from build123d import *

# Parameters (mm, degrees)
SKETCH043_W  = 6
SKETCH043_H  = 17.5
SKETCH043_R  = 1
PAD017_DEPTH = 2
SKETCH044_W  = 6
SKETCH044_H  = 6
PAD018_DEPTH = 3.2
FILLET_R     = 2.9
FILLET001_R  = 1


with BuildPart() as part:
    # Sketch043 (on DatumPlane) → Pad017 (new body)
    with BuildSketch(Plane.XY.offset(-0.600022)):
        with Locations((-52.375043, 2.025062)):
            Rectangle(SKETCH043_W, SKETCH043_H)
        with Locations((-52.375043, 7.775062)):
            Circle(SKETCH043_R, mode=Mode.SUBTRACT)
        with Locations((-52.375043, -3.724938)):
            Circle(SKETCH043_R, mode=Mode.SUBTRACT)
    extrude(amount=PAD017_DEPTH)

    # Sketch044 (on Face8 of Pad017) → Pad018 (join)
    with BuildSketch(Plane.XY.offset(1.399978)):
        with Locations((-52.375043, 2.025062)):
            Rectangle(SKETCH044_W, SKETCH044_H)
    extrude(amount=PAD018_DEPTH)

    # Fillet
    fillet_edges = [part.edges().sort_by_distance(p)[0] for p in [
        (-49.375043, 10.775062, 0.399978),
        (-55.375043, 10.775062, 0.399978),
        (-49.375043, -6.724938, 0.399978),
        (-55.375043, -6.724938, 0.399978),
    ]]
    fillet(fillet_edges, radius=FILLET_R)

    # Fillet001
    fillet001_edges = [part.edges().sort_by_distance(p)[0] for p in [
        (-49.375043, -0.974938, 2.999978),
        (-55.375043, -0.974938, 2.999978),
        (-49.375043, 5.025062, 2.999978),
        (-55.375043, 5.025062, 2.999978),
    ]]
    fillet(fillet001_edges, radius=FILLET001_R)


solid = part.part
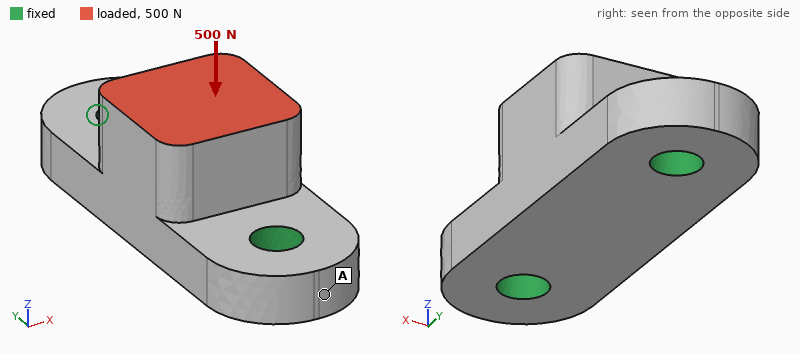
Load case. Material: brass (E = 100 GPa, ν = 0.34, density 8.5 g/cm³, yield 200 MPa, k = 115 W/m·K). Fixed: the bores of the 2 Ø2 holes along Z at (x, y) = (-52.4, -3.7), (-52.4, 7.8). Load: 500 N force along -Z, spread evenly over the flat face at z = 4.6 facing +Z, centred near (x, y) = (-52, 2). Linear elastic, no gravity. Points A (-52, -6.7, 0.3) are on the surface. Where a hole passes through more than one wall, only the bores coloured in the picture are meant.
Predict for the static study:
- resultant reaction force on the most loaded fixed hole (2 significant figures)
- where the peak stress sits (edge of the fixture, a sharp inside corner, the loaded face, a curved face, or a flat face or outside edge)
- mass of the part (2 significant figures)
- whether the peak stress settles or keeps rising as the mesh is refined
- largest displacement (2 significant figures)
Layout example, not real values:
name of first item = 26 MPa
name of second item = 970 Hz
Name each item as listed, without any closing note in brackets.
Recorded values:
resultant reaction force on the most loaded fixed hole = 270 N
where the peak stress sits = edge of the fixture
mass of the part = 2.5 g
whether the peak stress settles or keeps rising as the mesh is refined = keeps rising
largest displacement = 4.6 µm
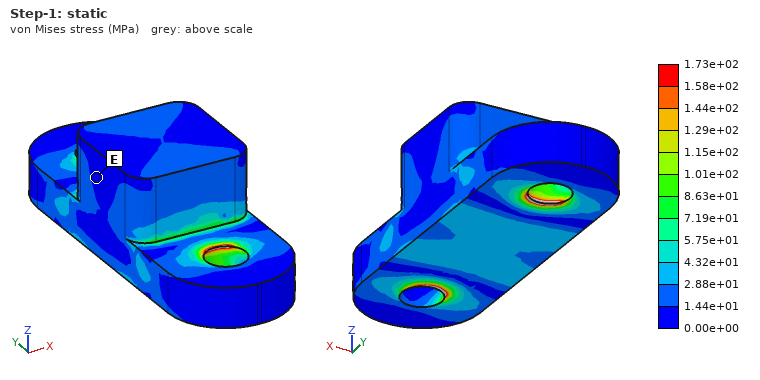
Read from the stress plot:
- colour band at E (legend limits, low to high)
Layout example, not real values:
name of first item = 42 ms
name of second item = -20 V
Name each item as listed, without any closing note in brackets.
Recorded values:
colour band at E = 0.00e+00 to 1.44e+01 MPa
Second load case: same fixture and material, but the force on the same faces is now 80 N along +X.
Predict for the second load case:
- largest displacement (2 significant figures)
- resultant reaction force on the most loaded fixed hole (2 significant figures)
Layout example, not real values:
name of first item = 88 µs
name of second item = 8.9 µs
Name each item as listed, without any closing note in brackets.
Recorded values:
largest displacement = 5.0 µm
resultant reaction force on the most loaded fixed hole = 40 N
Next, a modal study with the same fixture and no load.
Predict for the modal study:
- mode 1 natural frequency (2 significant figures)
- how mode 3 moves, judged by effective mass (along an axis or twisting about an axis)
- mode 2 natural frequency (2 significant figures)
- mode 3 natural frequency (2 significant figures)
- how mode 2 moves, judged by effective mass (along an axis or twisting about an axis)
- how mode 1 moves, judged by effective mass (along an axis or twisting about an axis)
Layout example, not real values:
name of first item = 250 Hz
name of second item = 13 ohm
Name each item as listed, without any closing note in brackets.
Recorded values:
mode 1 natural frequency = 27 kHz
how mode 3 moves, judged by effective mass = along Y
mode 2 natural frequency = 43 kHz
mode 3 natural frequency = 59 kHz
how mode 2 moves, judged by effective mass = along Z
how mode 1 moves, judged by effective mass = along X
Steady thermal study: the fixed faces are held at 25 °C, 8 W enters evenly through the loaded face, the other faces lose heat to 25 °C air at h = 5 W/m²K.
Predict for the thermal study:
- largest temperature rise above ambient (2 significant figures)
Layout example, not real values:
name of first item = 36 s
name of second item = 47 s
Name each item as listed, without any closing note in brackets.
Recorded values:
largest temperature rise above ambient = 17 K
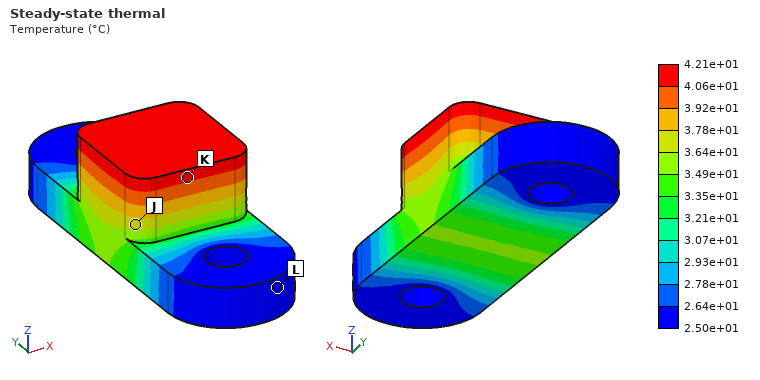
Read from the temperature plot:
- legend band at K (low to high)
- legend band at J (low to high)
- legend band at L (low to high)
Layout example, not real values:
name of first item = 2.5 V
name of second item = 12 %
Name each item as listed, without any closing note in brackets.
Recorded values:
legend band at K = 4.06e+01 to 4.21e+01 °C
legend band at J = 3.64e+01 to 3.78e+01 °C
legend band at L = 2.50e+01 to 2.64e+01 °C
